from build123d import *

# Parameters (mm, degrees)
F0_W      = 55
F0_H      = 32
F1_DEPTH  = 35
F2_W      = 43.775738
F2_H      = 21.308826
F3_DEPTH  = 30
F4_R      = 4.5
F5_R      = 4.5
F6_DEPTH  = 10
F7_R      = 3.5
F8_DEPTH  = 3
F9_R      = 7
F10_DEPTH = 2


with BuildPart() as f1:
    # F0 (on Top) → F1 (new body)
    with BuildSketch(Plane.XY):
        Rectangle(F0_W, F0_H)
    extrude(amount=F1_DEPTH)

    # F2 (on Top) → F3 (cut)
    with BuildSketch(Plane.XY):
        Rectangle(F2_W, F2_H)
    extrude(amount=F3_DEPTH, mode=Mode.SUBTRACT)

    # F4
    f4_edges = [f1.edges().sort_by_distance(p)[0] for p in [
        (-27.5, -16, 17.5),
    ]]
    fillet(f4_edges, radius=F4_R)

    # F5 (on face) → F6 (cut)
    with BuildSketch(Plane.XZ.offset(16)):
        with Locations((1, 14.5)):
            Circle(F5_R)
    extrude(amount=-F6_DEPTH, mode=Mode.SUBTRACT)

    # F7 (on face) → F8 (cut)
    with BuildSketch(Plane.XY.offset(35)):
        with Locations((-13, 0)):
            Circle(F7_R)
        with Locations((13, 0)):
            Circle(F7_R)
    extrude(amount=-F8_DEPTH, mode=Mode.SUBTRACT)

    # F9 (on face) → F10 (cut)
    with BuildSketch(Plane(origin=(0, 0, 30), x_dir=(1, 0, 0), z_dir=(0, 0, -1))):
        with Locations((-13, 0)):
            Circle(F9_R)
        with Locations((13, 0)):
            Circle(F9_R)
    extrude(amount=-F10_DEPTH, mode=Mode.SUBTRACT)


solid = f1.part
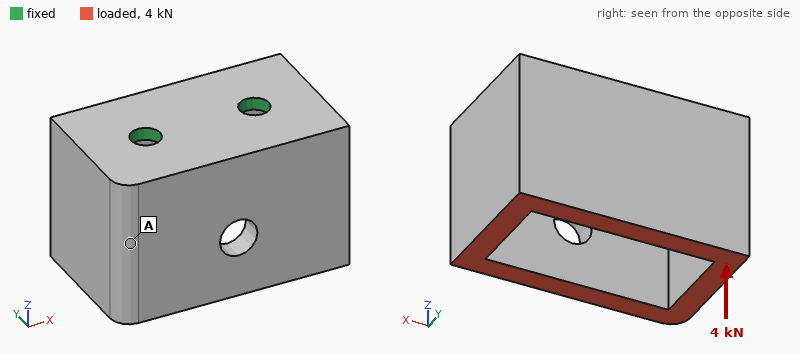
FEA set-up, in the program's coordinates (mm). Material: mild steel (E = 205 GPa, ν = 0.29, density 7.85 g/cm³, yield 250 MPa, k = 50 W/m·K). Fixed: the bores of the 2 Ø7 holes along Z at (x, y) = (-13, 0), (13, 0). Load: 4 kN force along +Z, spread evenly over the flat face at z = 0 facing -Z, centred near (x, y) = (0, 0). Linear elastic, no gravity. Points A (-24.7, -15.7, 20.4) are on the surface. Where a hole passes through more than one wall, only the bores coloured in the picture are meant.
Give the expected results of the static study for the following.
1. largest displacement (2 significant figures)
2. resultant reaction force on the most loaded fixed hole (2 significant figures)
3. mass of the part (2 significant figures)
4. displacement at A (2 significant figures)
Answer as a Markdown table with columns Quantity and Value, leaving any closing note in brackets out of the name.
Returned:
| Quantity | Value |
|---|---|
| largest displacement | 6.6 µm |
| resultant reaction force on the most loaded fixed hole | 2.0 kN |
| mass of the part | 250 g |
| displacement at A | 5.3 µm |
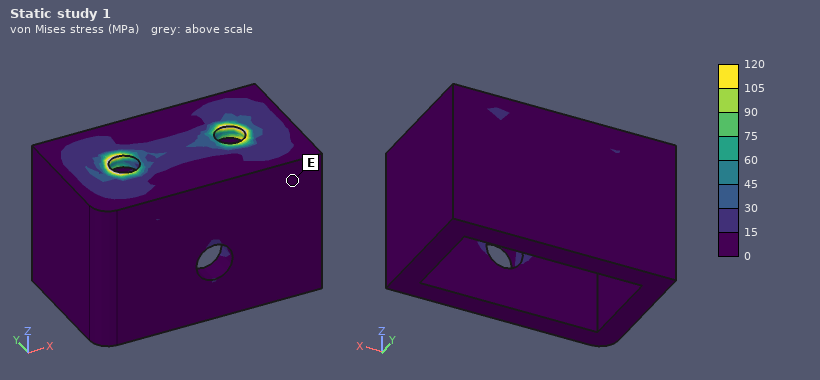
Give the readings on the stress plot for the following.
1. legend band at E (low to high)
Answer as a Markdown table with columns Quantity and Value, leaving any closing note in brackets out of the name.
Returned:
| Quantity | Value |
|---|---|
| legend band at E | 0 to 15 MPa |
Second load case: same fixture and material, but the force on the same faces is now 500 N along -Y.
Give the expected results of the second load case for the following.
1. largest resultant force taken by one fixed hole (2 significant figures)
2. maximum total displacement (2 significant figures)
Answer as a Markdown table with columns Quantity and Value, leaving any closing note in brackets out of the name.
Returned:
| Quantity | Value |
|---|---|
| largest resultant force taken by one fixed hole | 250 N |
| maximum total displacement | 32 µm |
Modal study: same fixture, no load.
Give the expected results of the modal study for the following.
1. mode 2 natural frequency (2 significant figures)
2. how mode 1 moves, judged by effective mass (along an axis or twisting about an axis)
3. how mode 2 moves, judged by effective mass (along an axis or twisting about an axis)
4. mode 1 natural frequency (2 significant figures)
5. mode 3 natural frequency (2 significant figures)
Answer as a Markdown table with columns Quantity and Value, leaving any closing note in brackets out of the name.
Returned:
| Quantity | Value |
|---|---|
| mode 2 natural frequency | 4900 Hz |
| how mode 1 moves, judged by effective mass | along Y |
| how mode 2 moves, judged by effective mass | along X |
| mode 1 natural frequency | 2200 Hz |
| mode 3 natural frequency | 5900 Hz |
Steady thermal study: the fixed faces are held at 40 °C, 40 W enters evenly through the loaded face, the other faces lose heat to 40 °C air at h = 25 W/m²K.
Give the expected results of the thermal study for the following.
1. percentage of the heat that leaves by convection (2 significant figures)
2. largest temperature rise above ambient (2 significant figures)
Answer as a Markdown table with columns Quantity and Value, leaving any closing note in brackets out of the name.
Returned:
| Quantity | Value |
|---|---|
| percentage of the heat that leaves by convection | 23 % |
| largest temperature rise above ambient | 49 K |
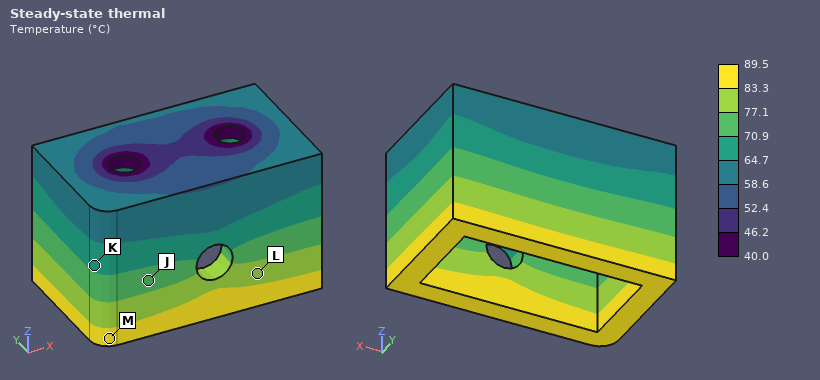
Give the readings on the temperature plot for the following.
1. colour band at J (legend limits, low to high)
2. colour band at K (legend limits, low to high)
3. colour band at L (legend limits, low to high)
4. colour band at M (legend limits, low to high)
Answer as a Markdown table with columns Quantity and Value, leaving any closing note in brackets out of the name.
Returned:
| Quantity | Value |
|---|---|
| colour band at J | 70.9 to 77.1 °C |
| colour band at K | 64.7 to 70.9 °C |
| colour band at L | 77.1 to 83.3 °C |
| colour band at M | 83.3 to 89.5 °C |
